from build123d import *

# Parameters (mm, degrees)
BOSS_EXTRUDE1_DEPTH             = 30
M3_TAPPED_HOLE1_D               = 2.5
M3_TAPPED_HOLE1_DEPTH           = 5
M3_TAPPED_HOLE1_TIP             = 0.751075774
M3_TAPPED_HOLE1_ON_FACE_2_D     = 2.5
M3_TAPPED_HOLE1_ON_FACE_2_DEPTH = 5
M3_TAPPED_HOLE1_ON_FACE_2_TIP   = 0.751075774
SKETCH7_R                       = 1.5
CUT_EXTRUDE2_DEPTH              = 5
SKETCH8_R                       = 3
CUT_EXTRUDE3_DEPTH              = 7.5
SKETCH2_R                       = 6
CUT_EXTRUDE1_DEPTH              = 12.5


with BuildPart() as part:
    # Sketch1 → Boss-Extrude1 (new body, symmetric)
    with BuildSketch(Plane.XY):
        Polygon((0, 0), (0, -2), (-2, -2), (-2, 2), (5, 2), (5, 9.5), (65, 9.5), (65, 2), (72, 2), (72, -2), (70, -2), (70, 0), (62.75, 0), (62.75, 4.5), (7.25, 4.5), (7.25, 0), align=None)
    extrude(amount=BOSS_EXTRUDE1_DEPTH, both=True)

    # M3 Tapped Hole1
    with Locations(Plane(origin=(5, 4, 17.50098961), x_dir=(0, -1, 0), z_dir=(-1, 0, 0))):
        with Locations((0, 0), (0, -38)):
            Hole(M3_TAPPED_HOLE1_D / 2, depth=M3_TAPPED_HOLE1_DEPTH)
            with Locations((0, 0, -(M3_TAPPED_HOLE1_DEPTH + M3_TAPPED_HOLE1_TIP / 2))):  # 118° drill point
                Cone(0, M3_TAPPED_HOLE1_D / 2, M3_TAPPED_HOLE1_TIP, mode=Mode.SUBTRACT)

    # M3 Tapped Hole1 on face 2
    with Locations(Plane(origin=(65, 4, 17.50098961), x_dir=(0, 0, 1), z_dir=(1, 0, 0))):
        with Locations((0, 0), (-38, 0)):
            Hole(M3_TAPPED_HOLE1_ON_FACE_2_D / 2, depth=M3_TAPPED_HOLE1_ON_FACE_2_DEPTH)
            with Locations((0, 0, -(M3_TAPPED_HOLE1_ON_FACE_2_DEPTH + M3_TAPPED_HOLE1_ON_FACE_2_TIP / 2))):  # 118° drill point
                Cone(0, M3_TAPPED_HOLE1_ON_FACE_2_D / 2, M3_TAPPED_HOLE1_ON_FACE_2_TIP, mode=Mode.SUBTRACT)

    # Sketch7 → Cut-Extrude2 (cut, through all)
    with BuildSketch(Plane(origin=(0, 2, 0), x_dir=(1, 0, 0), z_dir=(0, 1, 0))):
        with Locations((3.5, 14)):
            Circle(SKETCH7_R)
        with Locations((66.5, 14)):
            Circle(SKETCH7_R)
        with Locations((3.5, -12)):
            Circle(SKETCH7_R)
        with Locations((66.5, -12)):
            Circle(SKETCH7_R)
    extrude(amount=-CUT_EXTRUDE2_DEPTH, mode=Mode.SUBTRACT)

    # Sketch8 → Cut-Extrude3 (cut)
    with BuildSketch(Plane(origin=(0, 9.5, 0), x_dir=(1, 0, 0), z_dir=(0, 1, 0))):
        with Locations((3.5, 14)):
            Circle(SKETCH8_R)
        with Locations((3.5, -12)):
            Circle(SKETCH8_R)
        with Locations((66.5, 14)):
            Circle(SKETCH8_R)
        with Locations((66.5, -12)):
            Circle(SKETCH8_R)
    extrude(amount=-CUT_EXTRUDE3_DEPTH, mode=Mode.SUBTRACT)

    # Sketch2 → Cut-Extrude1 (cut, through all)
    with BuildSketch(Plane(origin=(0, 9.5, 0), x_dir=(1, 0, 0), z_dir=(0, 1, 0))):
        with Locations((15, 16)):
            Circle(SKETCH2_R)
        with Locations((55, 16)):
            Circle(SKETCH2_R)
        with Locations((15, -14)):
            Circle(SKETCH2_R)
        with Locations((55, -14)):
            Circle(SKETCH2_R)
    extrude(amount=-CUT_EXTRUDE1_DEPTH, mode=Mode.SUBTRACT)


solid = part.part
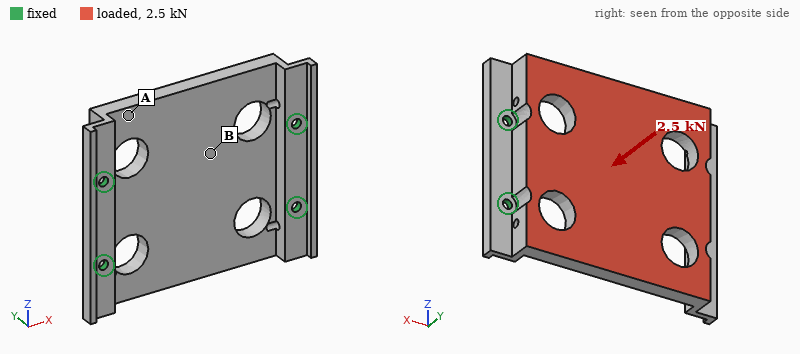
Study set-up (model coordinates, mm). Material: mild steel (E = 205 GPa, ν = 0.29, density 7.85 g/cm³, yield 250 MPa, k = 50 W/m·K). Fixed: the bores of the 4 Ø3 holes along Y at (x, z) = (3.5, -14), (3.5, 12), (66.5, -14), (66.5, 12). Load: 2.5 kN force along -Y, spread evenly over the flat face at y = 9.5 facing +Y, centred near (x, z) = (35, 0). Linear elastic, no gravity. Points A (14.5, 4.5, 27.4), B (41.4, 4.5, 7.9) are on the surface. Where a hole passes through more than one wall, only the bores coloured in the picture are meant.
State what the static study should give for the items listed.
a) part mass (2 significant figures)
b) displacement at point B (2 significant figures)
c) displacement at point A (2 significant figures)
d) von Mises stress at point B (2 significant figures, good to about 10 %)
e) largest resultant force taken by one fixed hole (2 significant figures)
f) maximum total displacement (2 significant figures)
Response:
150 g
26 µm
19 µm
32 MPa
1.1 kN
37 µm
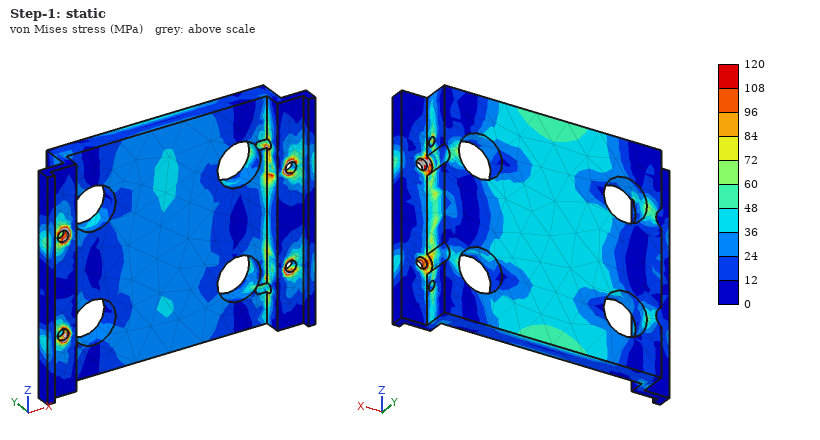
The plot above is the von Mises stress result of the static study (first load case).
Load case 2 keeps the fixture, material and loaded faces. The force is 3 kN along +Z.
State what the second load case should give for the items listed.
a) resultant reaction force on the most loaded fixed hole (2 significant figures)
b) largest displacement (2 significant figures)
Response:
960 N
18 µm
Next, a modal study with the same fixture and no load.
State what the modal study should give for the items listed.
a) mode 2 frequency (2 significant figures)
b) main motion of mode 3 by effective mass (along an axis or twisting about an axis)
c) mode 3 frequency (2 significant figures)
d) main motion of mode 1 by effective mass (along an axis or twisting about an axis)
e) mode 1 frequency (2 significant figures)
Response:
4900 Hz
along X
7400 Hz
along Y
4500 Hz
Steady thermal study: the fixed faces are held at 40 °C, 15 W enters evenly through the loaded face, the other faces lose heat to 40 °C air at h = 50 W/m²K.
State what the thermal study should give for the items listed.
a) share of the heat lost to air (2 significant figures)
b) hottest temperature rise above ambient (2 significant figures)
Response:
33 %
20 K
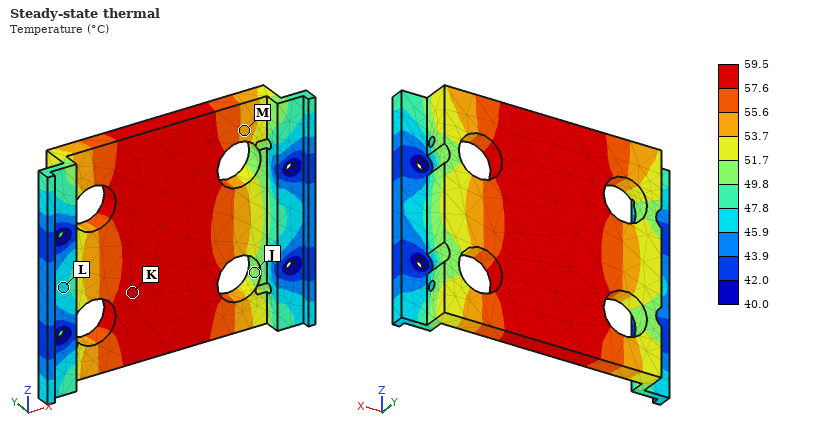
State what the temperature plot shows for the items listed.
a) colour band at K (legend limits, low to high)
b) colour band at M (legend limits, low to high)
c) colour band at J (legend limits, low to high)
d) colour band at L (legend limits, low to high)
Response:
57.6 to 59.5 °C
53.7 to 55.6 °C
49.8 to 51.7 °C
45.9 to 47.8 °C
